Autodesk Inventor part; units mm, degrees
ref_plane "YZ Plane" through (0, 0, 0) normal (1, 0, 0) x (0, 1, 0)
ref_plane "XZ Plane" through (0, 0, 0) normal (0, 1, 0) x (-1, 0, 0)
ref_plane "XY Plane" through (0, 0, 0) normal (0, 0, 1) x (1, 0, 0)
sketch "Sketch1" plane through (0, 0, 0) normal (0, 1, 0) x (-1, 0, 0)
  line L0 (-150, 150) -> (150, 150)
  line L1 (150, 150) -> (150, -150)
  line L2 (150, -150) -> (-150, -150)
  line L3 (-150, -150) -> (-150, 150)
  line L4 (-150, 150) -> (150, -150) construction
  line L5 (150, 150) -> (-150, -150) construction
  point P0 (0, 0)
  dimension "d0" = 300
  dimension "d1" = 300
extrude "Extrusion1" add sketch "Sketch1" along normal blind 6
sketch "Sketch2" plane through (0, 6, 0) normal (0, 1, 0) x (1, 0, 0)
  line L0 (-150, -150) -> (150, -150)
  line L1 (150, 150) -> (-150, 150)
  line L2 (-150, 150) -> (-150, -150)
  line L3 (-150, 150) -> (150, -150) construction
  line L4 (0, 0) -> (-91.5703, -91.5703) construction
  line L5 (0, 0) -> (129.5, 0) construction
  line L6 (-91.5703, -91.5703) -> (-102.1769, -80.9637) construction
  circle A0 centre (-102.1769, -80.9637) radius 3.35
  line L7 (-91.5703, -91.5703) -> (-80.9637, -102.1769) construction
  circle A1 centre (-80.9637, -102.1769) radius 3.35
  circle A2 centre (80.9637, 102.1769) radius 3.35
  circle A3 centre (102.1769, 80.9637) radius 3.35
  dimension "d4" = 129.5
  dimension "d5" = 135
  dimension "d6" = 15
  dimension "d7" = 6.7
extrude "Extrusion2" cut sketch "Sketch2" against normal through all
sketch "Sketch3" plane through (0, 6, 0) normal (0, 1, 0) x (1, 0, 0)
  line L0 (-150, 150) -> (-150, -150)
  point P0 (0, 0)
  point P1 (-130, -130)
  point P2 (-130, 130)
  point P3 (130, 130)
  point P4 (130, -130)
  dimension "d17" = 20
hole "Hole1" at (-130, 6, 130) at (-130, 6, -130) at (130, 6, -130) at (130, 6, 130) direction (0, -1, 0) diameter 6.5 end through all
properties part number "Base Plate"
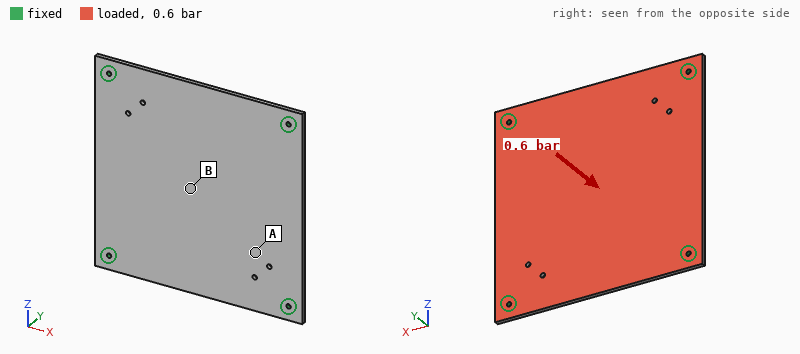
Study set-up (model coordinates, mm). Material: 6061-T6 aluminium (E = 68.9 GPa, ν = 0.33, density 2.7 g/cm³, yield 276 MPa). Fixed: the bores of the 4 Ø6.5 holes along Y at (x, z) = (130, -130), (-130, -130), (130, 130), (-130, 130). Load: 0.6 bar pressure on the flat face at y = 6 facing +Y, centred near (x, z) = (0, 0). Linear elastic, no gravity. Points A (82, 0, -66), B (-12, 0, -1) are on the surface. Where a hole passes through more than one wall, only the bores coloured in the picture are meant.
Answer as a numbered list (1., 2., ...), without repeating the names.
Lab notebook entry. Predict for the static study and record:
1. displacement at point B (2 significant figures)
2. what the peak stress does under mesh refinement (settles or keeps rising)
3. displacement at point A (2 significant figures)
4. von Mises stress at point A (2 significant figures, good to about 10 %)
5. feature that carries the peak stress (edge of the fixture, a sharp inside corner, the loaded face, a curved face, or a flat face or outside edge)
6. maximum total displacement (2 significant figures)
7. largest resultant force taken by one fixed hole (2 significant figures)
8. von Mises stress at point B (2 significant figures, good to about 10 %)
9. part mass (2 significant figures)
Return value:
1. 1.7 mm
2. keeps rising
3. 1.0 mm
4. 21 MPa
5. edge of the fixture
6. 1.7 mm
7. 1.3 kN
8. 40 MPa
9. 1.5 kg
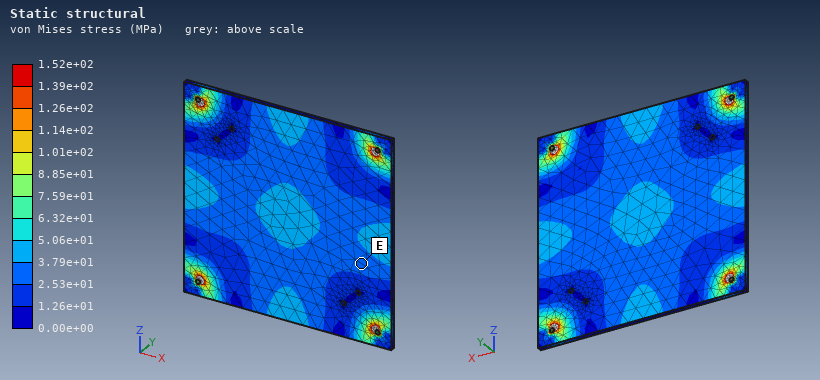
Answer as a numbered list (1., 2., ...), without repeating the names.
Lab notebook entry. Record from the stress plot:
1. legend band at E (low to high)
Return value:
1. 2.53e+01 to 3.79e+01 MPa
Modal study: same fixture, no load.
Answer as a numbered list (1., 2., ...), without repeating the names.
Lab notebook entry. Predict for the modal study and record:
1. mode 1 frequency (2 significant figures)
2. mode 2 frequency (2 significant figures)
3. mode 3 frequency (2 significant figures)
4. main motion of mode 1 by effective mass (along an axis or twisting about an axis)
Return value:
1. 280 Hz
2. 490 Hz
3. 490 Hz
4. along Y
